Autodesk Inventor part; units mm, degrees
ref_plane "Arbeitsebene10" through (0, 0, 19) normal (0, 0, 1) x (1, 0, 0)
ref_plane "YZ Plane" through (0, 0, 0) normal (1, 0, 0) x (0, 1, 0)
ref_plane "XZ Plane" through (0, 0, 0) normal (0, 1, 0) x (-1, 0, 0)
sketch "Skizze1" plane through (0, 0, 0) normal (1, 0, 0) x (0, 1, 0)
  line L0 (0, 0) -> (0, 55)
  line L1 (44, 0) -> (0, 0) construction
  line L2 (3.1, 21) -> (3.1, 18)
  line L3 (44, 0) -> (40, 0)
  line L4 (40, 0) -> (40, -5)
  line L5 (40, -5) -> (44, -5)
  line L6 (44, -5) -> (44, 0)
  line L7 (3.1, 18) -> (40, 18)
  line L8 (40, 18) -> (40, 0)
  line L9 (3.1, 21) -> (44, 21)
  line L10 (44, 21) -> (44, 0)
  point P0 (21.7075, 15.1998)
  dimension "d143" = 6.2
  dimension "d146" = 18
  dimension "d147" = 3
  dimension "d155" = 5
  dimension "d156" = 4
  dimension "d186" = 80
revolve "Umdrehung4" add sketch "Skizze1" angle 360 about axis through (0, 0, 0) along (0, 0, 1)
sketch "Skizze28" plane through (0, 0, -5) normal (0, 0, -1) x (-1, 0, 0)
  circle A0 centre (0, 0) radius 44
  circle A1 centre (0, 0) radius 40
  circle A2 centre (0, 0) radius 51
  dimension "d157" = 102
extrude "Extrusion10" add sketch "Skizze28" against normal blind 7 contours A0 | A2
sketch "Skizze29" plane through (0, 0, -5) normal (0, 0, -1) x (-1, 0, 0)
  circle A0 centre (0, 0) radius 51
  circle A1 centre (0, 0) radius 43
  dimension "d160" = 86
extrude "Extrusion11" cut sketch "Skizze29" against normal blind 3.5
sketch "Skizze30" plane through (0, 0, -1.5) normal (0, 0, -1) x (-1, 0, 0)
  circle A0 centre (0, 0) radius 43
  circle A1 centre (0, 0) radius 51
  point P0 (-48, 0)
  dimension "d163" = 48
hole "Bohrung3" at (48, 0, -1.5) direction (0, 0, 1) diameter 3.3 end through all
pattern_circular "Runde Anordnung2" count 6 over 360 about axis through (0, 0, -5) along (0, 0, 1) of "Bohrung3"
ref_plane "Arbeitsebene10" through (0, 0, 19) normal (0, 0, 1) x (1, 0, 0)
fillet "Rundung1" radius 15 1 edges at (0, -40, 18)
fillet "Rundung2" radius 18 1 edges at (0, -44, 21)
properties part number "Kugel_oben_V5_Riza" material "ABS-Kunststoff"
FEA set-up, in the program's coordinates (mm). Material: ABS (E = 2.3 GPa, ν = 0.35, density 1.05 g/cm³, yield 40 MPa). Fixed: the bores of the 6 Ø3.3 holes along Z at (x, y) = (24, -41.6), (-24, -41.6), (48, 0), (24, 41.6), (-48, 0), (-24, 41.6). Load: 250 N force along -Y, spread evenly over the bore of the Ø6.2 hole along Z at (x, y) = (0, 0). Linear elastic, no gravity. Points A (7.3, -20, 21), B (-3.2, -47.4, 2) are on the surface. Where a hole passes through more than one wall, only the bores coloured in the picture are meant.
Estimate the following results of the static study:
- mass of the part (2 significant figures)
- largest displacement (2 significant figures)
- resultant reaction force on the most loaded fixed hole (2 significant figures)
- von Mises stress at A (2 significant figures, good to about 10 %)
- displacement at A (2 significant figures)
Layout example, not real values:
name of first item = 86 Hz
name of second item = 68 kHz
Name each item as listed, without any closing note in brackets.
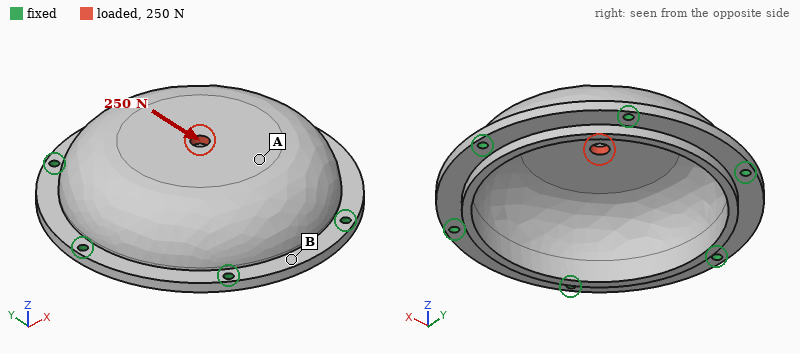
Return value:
mass of the part = 44 g
largest displacement = 63 µm
resultant reaction force on the most loaded fixed hole = 55 N
von Mises stress at A = 1.4 MPa
displacement at A = 48 µm
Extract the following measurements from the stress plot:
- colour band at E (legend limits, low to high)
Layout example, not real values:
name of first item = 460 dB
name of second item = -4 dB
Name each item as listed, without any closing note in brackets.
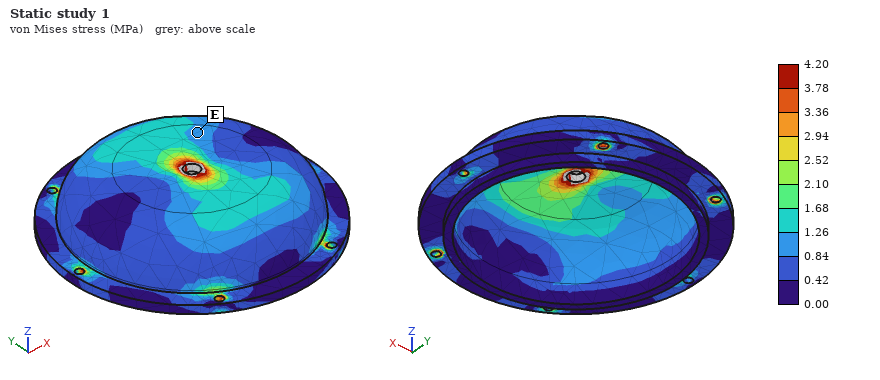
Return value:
colour band at E = 0.84 to 1.26 MPa
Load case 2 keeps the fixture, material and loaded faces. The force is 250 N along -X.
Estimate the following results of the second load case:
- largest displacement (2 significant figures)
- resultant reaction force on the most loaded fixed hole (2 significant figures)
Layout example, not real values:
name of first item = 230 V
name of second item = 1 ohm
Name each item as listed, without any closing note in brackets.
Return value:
largest displacement = 63 µm
resultant reaction force on the most loaded fixed hole = 52 N
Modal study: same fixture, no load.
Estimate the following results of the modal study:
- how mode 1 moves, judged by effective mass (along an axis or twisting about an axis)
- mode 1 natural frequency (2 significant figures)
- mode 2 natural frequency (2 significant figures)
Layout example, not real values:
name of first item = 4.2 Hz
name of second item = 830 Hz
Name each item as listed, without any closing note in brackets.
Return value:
how mode 1 moves, judged by effective mass = along Z
mode 1 natural frequency = 1800 Hz
mode 2 natural frequency = 3100 Hz
